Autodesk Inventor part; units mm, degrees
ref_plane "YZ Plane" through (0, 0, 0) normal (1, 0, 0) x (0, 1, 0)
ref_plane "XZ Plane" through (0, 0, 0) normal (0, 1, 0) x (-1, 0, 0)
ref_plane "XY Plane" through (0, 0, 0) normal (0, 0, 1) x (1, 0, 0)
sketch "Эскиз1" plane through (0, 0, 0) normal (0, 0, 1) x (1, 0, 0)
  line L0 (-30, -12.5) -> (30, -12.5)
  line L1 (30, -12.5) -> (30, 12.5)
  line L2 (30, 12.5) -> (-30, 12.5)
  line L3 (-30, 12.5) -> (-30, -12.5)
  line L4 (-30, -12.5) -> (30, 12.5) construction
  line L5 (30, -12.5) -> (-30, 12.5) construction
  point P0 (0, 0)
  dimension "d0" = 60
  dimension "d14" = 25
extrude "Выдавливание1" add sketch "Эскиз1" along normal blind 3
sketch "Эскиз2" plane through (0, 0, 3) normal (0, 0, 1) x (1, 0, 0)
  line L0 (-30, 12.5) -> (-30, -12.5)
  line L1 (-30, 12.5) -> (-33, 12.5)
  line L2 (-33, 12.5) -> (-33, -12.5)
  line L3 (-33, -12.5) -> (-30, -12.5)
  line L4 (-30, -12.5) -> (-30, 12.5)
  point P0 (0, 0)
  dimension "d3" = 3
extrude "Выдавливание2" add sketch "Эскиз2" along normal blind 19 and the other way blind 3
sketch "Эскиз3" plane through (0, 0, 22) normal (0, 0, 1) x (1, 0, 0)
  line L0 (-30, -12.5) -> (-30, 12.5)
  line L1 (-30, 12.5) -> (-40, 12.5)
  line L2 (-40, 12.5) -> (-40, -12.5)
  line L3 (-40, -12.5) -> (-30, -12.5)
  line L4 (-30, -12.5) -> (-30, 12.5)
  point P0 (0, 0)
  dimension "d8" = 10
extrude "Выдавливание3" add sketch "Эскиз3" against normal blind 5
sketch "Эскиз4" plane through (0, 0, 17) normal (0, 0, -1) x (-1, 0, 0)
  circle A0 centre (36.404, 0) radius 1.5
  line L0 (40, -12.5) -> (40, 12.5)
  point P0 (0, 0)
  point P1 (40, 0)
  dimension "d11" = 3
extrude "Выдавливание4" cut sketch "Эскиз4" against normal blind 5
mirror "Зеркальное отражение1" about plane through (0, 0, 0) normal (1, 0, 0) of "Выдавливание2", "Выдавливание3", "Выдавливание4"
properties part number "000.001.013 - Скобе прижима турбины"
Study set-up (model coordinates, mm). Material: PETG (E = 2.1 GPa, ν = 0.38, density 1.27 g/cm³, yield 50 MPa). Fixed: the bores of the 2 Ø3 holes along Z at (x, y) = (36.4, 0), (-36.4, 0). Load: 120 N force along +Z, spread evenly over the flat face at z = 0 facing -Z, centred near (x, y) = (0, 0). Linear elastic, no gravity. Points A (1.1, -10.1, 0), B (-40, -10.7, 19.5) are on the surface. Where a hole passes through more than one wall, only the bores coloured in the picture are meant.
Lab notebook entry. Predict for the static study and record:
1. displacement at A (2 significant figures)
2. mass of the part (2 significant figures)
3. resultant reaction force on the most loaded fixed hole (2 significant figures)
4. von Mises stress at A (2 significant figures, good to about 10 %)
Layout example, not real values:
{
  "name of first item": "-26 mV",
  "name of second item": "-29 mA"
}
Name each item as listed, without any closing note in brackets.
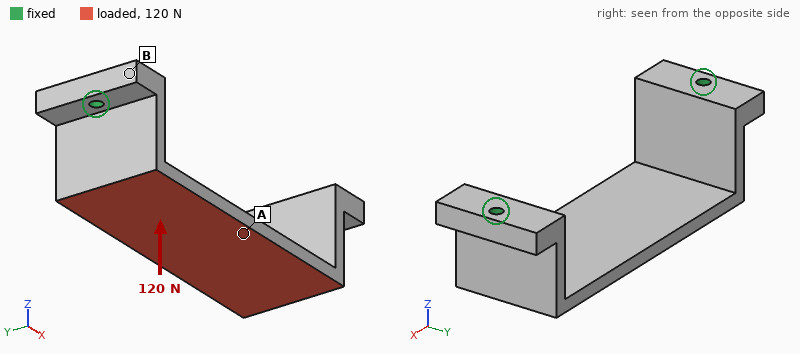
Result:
{
  "displacement at A": "0.86 mm",
  "mass of the part": "12 g",
  "resultant reaction force on the most loaded fixed hole": "76 N",
  "von Mises stress at A": "9.9 MPa"
}
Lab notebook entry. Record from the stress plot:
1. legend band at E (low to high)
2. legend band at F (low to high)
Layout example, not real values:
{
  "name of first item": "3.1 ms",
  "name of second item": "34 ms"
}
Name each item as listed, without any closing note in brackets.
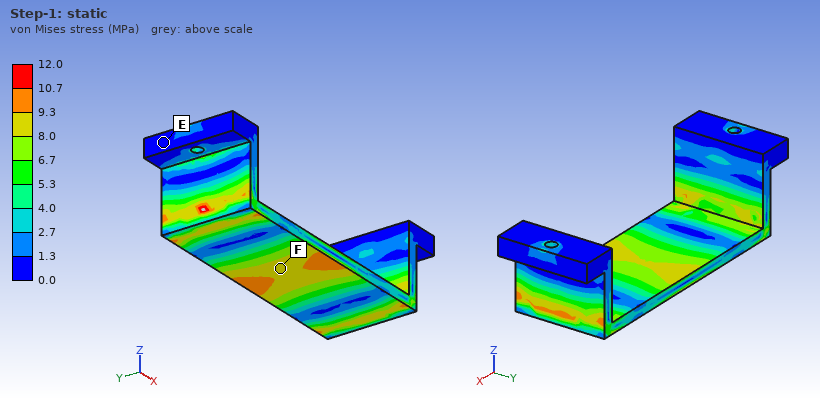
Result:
{
  "legend band at E": "0.0 to 1.3 MPa",
  "legend band at F": "8.0 to 9.3 MPa"
}
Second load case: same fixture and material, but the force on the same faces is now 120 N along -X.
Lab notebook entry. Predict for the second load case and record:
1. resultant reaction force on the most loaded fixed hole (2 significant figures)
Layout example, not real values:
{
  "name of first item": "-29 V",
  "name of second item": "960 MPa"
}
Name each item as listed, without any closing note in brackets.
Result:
{
  "resultant reaction force on the most loaded fixed hole": "62 N"
}
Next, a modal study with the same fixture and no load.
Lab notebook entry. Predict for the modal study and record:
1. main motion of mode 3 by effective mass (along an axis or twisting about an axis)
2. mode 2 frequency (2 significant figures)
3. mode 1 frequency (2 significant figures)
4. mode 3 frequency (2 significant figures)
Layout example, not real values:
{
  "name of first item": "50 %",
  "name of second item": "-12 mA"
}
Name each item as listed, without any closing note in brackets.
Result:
{
  "main motion of mode 3 by effective mass": "along Y",
  "mode 2 frequency": "880 Hz",
  "mode 1 frequency": "860 Hz",
  "mode 3 frequency": "1100 Hz"
}
